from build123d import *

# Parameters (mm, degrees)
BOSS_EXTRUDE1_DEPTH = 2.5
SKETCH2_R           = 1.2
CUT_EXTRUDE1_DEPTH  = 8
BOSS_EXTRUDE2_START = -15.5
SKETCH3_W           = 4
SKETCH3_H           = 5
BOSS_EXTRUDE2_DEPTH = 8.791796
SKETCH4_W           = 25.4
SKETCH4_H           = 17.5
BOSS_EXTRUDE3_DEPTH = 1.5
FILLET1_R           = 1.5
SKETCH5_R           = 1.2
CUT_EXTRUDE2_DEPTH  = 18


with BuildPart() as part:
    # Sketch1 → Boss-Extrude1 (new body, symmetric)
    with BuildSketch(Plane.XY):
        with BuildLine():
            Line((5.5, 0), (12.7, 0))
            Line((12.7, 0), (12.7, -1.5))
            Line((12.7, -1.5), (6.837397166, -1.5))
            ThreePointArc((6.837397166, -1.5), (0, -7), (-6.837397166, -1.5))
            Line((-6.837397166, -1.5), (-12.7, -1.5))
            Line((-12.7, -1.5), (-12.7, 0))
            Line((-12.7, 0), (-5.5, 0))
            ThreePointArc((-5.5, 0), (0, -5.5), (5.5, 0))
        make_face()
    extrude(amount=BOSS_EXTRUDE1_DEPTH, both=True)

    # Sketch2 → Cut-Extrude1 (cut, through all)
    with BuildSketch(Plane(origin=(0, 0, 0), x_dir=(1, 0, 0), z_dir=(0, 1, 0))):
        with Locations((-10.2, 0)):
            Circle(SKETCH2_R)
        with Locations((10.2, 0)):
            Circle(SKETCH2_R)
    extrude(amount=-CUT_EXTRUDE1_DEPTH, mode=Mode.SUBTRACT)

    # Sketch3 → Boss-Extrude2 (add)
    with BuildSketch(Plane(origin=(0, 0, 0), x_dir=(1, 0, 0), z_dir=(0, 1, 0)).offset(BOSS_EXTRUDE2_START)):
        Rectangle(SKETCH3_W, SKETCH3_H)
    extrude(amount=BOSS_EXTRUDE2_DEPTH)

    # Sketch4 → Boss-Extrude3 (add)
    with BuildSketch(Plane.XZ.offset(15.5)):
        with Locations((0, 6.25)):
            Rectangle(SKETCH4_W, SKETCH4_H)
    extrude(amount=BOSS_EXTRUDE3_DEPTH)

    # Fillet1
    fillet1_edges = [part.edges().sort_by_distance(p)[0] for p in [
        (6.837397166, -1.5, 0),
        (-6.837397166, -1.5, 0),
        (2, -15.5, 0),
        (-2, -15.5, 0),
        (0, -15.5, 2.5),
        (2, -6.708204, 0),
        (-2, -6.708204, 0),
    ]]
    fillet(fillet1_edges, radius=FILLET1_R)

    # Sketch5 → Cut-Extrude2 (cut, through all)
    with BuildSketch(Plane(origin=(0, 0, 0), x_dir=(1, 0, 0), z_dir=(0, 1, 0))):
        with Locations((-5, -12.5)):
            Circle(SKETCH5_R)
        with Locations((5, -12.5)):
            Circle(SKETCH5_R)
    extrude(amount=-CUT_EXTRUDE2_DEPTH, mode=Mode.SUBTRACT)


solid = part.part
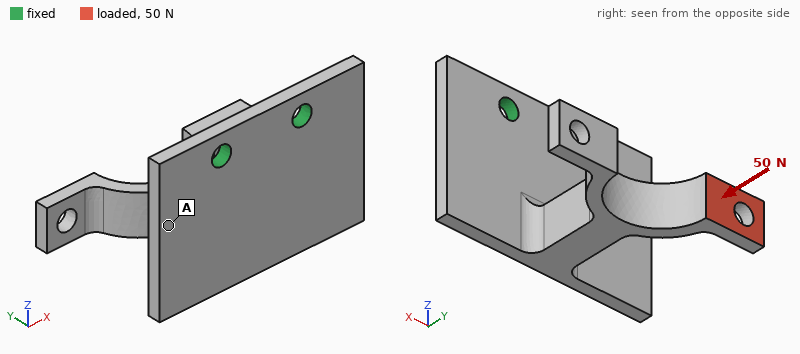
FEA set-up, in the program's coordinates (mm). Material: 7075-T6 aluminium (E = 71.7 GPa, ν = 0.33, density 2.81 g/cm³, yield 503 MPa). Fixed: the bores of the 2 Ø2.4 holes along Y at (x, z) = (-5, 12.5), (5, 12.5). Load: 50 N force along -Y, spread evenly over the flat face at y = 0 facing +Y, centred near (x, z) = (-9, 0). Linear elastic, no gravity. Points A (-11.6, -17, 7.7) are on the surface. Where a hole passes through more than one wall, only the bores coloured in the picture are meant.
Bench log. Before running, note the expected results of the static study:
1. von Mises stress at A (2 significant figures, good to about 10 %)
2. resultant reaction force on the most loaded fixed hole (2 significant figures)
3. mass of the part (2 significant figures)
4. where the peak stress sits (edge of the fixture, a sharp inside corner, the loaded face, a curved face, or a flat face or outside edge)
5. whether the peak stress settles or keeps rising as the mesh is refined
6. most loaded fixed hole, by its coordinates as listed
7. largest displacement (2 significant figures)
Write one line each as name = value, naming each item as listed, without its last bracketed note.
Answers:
von Mises stress at A = 40 MPa
resultant reaction force on the most loaded fixed hole = 62 N
mass of the part = 3.0 g
where the peak stress sits = edge of the fixture
whether the peak stress settles or keeps rising as the mesh is refined = keeps rising
most loaded fixed hole, by its coordinates as listed = (-5, 12.5)
largest displacement = 0.39 mm
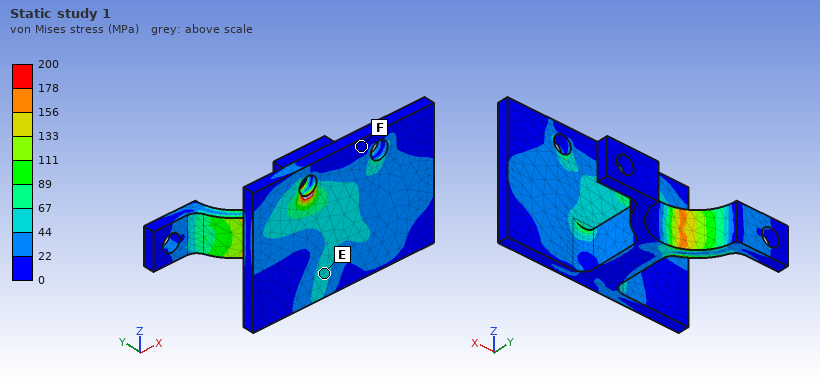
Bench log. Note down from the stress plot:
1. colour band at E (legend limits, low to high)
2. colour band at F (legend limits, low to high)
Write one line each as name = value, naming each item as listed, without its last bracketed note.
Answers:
colour band at E = 44 to 67 MPa
colour band at F = 0 to 22 MPa
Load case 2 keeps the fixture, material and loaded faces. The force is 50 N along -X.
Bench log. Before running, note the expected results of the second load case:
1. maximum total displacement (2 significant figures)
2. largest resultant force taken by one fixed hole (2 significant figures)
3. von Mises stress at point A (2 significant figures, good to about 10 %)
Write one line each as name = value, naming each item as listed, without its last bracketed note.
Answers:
maximum total displacement = 0.36 mm
largest resultant force taken by one fixed hole = 88 N
von Mises stress at point A = 19 MPa
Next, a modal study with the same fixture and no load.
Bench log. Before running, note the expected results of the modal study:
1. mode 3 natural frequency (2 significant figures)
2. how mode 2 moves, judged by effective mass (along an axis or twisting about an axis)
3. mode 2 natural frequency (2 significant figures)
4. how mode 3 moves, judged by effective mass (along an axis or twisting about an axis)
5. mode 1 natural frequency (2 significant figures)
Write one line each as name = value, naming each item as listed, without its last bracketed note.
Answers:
mode 3 natural frequency = 6900 Hz
how mode 2 moves, judged by effective mass = along X
mode 2 natural frequency = 3200 Hz
how mode 3 moves, judged by effective mass = along Y
mode 1 natural frequency = 2200 Hz
